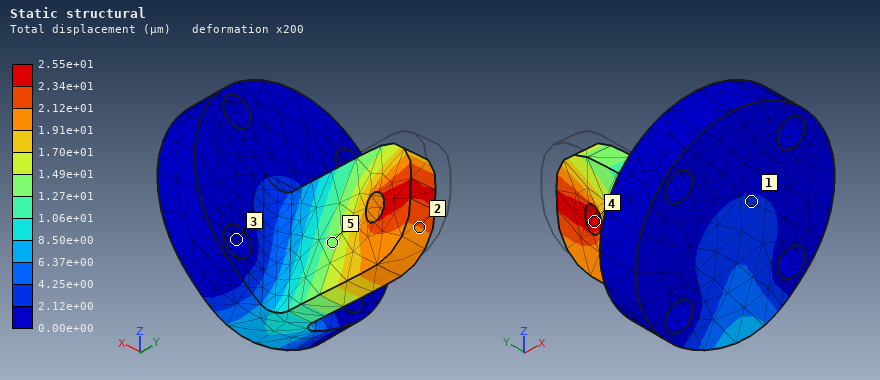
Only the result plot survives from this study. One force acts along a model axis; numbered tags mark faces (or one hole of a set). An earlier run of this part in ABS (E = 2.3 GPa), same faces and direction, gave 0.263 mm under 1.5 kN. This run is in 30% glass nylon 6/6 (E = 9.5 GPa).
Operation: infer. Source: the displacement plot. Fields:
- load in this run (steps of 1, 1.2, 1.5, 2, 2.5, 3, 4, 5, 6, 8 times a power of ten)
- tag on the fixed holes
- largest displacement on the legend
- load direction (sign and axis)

600 N
3
2.55e+01 µm
-Y
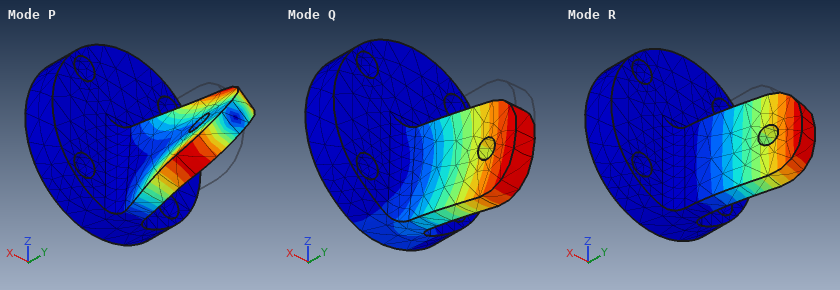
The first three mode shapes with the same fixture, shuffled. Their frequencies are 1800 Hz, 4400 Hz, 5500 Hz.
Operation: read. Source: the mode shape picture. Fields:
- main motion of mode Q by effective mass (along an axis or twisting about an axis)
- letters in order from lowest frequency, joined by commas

along Z
R, Q, P
